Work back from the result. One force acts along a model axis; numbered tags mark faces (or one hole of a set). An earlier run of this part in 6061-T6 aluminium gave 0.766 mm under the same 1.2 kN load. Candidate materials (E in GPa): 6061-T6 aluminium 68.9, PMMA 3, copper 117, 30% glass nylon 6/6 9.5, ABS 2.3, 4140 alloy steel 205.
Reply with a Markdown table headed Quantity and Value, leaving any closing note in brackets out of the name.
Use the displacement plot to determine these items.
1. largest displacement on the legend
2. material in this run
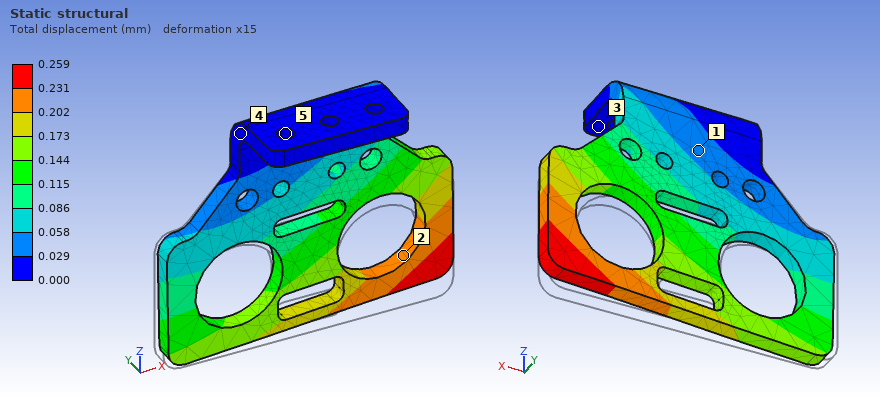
| Quantity | Value |
|---|---|
| largest displacement on the legend | 0.259 mm |
| material in this run | 4140 alloy steel |
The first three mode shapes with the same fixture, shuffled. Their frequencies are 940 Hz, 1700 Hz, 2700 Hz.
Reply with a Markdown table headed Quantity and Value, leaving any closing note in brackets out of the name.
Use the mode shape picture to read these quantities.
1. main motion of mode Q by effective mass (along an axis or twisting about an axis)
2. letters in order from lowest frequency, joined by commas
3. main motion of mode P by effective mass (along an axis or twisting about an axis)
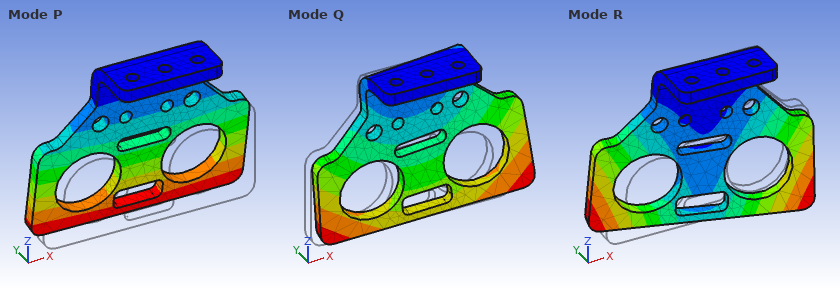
| Quantity | Value |
|---|---|
| main motion of mode Q by effective mass | along X |
| letters in order from lowest frequency, joined by commas | P, R, Q |
| main motion of mode P by effective mass | along Y |
